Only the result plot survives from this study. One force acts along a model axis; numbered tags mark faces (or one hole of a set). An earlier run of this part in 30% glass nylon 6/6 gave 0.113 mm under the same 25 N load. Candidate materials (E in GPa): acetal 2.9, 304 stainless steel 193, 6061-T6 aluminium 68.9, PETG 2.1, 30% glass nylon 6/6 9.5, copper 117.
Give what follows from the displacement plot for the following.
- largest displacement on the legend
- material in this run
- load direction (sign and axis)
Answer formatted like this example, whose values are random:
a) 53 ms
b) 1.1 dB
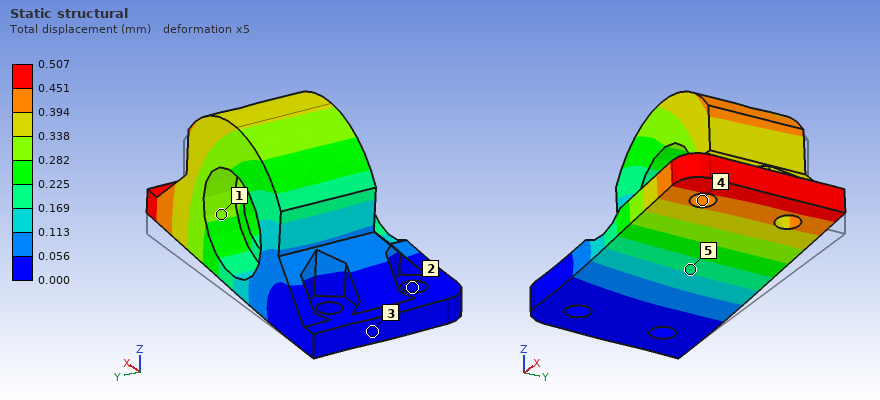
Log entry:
a) 0.507 mm
b) PETG
c) +Z
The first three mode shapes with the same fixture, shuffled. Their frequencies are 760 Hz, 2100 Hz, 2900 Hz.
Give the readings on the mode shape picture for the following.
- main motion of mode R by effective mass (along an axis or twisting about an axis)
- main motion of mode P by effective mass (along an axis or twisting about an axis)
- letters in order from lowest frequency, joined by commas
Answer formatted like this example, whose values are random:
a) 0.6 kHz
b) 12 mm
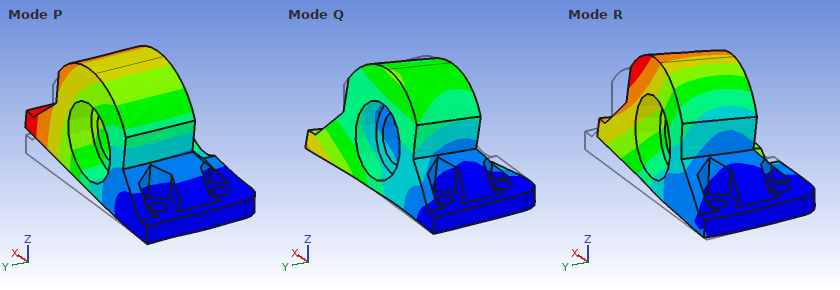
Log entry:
a) along Y
b) along Z
c) P, R, Q
